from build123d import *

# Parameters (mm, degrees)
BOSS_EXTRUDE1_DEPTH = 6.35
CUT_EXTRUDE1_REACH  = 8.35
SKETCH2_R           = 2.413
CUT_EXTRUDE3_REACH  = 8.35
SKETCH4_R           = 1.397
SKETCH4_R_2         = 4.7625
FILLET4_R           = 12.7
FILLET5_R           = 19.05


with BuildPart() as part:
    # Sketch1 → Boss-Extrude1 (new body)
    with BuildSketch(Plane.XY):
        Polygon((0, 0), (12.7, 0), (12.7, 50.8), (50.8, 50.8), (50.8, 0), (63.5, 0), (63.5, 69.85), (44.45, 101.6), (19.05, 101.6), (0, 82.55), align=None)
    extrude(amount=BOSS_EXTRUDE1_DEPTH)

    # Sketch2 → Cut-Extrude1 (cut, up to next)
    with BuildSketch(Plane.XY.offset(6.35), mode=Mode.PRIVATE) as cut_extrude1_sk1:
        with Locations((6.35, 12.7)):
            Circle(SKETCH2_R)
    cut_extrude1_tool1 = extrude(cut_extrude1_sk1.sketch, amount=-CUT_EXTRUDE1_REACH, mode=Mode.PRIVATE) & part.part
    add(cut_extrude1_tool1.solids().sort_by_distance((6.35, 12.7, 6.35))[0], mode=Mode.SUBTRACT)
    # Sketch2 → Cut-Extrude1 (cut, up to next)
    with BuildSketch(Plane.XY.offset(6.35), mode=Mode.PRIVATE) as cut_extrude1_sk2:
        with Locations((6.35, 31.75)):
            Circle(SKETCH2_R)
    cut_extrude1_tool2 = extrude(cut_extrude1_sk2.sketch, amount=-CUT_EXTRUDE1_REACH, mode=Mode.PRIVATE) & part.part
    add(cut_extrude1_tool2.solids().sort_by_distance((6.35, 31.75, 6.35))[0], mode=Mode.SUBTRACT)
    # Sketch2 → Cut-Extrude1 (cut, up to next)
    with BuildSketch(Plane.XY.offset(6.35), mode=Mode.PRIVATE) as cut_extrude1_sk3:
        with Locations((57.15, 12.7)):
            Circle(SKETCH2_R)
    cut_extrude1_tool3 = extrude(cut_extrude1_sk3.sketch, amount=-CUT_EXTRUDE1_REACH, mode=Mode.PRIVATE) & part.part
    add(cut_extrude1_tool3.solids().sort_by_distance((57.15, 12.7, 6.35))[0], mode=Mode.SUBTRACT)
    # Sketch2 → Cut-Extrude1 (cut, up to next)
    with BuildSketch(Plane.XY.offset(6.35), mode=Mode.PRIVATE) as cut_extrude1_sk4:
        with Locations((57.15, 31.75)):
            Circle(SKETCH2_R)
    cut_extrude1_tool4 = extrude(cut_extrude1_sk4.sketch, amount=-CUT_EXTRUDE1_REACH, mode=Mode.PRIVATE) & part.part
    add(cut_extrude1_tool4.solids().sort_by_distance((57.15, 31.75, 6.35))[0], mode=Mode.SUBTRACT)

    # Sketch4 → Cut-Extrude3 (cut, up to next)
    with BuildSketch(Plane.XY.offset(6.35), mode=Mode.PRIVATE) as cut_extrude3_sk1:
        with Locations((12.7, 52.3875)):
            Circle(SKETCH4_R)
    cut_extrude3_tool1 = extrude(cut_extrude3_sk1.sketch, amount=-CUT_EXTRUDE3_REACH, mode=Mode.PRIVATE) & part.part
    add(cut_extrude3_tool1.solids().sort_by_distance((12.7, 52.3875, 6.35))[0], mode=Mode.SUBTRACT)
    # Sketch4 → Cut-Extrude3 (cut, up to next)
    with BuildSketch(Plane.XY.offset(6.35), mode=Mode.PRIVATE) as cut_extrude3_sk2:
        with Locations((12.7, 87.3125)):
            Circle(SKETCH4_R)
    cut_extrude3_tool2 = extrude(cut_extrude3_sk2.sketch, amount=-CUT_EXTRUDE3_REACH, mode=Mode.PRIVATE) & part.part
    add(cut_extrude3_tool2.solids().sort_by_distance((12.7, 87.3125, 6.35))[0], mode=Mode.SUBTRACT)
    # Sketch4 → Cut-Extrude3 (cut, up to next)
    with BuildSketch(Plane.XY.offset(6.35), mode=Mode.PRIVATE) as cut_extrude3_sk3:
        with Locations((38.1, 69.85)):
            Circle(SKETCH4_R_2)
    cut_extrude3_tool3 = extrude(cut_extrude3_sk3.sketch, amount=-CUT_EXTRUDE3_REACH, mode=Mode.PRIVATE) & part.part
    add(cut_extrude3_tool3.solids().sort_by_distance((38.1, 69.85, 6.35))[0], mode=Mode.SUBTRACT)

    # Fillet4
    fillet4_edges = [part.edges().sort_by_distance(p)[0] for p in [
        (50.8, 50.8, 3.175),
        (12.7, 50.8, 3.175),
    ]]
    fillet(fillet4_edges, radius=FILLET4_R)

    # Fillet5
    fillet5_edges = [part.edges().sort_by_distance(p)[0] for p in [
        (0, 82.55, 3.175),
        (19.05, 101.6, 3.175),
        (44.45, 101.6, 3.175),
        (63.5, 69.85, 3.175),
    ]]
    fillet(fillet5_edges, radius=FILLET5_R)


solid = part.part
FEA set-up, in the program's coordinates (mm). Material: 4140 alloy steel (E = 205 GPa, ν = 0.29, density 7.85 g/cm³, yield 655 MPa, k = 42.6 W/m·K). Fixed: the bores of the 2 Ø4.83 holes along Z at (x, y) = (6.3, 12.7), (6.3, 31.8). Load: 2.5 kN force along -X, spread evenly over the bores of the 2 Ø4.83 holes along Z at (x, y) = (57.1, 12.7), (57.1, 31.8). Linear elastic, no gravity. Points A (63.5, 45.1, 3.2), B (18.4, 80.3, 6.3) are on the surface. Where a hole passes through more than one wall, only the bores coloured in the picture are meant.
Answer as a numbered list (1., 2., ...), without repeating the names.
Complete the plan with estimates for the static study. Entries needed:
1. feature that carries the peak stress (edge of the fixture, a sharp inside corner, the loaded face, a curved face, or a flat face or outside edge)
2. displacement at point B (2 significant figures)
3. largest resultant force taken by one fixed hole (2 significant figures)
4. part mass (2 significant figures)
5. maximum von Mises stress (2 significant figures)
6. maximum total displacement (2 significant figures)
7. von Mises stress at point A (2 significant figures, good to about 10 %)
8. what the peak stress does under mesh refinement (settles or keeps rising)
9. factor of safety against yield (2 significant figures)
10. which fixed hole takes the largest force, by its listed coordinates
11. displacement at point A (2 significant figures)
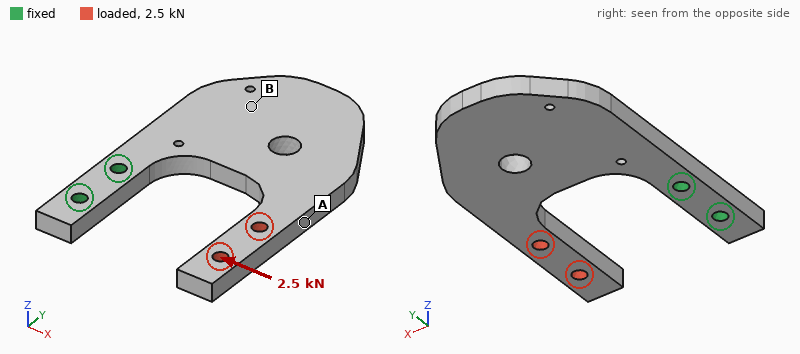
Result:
1. a curved face
2. 0.17 mm
3. 2.0 kN
4. 190 g
5. 360 MPa
6. 0.57 mm
7. 260 MPa
8. settles
9. 1.8
10. (6.3, 31.8)
11. 0.29 mm
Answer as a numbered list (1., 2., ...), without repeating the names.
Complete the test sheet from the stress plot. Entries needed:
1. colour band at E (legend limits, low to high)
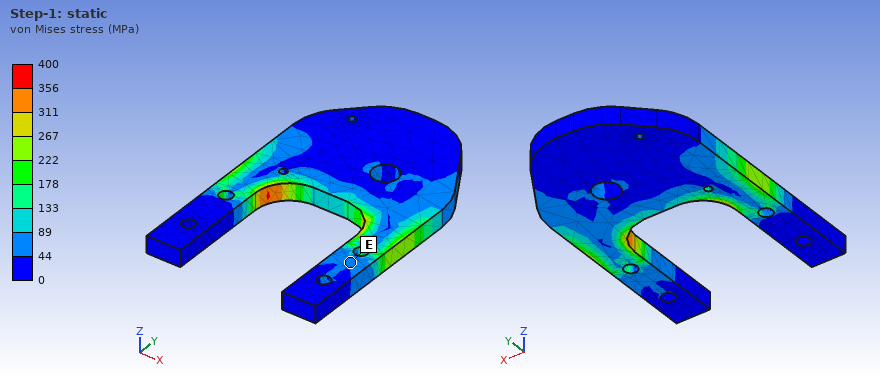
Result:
1. 44 to 89 MPa
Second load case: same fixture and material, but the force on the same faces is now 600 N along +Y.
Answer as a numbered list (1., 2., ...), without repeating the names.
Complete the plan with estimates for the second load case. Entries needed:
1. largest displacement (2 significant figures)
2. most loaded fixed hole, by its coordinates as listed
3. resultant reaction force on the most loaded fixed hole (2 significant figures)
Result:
1. 0.21 mm
2. (6.3, 31.8)
3. 830 N
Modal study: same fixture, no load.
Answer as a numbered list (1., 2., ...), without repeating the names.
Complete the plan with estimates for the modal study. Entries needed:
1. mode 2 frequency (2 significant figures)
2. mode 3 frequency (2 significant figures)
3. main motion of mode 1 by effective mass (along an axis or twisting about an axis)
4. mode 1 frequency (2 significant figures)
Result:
1. 650 Hz
2. 830 Hz
3. along Z
4. 510 Hz
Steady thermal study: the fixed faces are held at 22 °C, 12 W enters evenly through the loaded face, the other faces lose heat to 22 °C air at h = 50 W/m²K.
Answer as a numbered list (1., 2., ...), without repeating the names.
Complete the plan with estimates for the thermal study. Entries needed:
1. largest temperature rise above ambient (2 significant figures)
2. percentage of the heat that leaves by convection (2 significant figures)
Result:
1. 83 K
2. 90 %
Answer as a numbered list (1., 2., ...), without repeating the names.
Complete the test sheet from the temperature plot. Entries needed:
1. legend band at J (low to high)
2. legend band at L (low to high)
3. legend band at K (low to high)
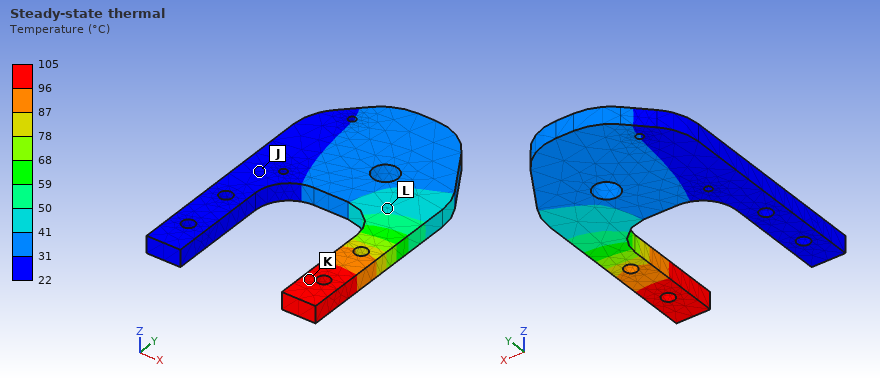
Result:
1. 22 to 31 °C
2. 41 to 50 °C
3. 96 to 105 °C
